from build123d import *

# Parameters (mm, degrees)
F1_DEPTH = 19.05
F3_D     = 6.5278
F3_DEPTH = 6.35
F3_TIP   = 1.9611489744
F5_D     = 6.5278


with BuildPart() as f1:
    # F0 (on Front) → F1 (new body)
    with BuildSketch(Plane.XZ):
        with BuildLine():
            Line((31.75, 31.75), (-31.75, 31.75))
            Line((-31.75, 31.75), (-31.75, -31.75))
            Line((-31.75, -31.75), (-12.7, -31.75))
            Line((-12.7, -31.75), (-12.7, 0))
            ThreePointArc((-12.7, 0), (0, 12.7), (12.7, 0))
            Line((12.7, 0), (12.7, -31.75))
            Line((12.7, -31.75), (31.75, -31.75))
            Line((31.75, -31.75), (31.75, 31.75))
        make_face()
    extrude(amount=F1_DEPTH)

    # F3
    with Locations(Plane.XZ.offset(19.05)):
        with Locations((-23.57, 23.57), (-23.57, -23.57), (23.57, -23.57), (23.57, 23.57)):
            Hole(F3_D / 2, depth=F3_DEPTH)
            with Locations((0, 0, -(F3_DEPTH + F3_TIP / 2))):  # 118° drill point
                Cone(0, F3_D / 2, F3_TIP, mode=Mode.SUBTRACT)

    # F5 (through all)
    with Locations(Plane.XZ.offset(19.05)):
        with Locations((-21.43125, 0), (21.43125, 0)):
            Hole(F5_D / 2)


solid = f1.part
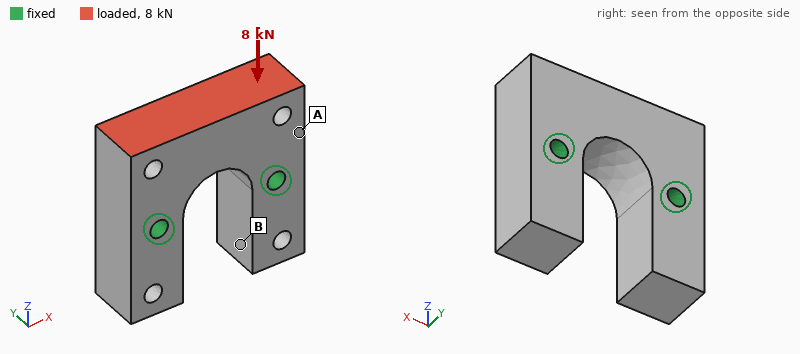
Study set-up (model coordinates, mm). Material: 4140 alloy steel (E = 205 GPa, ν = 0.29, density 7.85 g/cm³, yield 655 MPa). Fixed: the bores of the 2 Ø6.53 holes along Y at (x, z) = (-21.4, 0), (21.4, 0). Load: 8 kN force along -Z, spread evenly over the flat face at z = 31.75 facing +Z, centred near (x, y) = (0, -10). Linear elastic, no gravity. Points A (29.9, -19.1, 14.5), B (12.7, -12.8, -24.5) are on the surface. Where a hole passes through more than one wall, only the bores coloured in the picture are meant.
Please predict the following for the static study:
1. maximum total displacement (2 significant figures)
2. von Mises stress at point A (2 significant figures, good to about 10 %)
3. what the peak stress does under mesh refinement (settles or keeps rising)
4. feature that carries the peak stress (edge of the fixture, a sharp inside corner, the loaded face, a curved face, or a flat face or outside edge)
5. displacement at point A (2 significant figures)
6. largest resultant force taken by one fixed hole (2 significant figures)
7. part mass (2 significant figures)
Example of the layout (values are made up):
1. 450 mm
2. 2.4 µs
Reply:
1. 1.8 µm
2. 6.8 MPa
3. keeps rising
4. edge of the fixture
5. 0.69 µm
6. 4.1 kN
7. 430 g
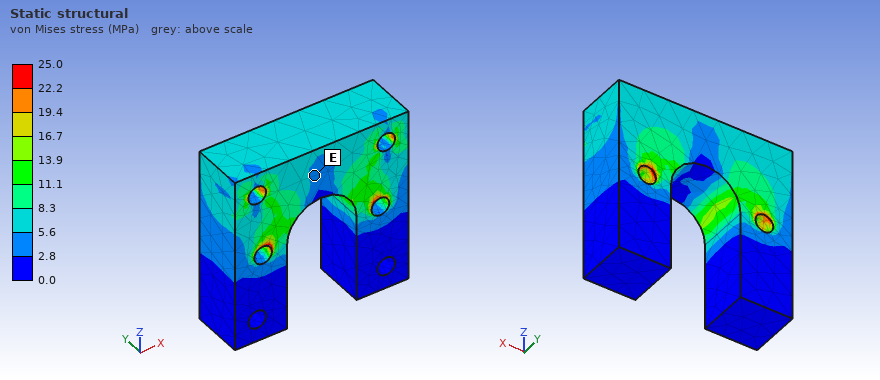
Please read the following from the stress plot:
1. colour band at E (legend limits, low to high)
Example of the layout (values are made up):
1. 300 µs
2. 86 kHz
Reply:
1. 2.8 to 5.6 MPa
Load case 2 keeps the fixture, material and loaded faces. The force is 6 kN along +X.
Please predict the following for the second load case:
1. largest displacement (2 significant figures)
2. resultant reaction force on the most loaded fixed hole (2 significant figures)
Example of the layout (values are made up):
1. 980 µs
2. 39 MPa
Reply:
1. 5.9 µm
2. 4.6 kN
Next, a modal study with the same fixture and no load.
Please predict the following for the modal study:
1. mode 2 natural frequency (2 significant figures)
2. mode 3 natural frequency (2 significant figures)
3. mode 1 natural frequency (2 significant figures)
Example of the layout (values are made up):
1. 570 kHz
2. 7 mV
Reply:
1. 11 kHz
2. 11 kHz
3. 10 kHz
